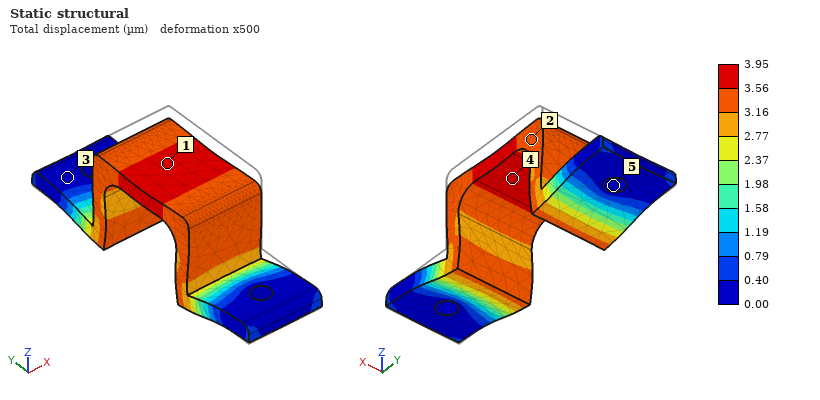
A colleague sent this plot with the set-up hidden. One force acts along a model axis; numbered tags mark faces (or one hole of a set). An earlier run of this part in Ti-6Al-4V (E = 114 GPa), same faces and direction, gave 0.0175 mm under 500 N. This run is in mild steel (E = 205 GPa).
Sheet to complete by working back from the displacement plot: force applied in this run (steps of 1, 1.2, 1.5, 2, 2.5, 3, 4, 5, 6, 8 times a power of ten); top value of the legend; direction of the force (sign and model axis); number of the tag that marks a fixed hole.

200 N
3.95 µm
-Z
5
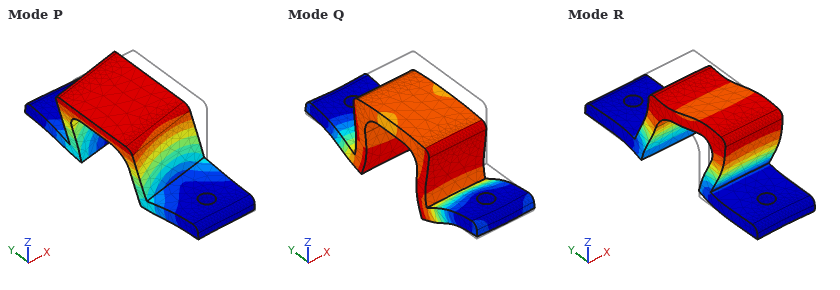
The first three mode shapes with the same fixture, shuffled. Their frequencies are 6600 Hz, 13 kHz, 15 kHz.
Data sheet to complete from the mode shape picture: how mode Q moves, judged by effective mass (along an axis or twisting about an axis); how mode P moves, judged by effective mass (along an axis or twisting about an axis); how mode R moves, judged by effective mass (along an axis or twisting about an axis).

along Z
along X
along Y
